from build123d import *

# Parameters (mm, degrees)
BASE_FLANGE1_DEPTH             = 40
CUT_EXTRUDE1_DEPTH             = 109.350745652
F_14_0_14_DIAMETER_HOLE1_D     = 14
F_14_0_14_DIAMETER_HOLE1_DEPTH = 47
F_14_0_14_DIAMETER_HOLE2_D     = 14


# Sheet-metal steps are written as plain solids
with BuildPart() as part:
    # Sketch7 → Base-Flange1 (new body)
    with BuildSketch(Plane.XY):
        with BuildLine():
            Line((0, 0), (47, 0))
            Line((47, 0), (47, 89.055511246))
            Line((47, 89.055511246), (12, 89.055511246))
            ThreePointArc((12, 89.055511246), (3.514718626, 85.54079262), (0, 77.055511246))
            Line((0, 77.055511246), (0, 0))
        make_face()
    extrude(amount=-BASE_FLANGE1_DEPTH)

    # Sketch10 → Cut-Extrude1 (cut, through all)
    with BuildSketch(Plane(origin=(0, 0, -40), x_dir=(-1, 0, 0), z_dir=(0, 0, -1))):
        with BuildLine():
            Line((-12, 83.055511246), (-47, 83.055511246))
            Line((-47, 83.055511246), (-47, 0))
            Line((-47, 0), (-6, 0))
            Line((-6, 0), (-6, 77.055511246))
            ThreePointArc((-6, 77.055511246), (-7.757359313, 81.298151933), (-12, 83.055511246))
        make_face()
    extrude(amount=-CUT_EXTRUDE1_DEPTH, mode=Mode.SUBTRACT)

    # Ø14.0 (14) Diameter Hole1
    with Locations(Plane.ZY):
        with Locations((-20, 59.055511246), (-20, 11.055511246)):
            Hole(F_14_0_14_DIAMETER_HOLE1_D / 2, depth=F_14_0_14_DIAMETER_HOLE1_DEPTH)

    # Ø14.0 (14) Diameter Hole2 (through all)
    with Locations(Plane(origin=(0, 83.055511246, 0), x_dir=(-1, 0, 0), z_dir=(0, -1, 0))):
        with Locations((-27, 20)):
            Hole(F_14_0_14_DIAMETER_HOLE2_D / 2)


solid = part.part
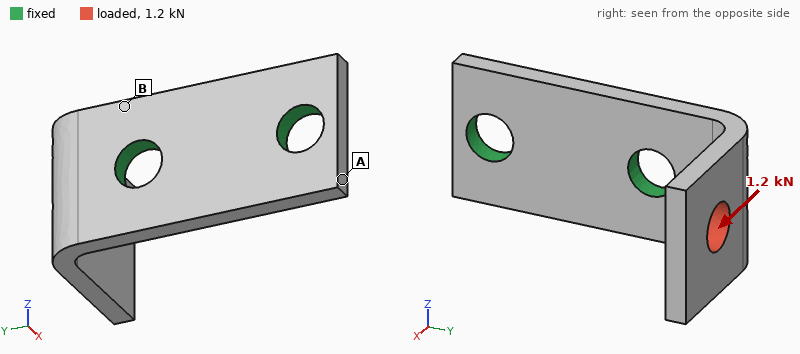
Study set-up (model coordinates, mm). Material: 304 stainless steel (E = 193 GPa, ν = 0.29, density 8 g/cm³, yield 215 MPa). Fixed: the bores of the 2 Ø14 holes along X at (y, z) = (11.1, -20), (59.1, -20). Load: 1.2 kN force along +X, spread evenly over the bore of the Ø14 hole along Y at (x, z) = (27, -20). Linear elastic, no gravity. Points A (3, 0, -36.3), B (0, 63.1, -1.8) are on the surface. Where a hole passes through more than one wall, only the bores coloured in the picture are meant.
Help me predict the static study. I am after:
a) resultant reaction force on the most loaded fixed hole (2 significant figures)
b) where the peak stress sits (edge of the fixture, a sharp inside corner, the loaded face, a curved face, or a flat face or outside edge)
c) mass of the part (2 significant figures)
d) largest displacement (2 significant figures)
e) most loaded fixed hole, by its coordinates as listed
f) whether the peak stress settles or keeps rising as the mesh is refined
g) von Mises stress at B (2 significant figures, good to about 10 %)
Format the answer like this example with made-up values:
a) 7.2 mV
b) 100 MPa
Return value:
a) 1.2 kN
b) edge of the fixture
c) 220 g
d) 0.11 mm
e) (59.1, -20)
f) keeps rising
g) 45 MPa
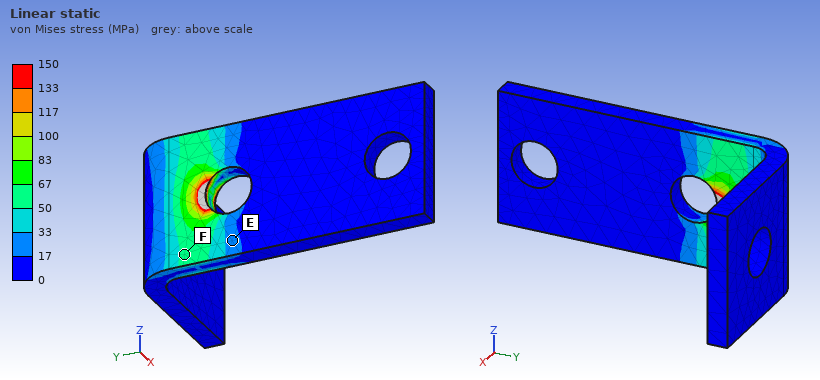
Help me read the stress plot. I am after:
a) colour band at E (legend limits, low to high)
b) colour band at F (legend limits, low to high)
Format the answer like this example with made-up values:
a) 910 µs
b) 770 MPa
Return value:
a) 17 to 33 MPa
b) 50 to 67 MPa
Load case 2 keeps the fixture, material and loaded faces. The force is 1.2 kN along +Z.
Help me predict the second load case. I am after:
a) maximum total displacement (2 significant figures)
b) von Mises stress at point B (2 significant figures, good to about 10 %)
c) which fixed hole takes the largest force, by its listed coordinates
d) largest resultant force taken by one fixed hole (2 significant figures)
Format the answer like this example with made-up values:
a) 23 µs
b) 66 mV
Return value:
a) 0.11 mm
b) 60 MPa
c) (59.1, -20)
d) 1.5 kN
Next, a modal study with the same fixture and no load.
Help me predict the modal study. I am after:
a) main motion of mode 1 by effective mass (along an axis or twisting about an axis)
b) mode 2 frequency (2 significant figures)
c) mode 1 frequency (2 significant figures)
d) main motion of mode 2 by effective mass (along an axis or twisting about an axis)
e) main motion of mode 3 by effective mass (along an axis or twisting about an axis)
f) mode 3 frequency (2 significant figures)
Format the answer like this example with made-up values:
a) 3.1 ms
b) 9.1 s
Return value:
a) along Y
b) 2200 Hz
c) 1500 Hz
d) along Z
e) along X
f) 4800 Hz
